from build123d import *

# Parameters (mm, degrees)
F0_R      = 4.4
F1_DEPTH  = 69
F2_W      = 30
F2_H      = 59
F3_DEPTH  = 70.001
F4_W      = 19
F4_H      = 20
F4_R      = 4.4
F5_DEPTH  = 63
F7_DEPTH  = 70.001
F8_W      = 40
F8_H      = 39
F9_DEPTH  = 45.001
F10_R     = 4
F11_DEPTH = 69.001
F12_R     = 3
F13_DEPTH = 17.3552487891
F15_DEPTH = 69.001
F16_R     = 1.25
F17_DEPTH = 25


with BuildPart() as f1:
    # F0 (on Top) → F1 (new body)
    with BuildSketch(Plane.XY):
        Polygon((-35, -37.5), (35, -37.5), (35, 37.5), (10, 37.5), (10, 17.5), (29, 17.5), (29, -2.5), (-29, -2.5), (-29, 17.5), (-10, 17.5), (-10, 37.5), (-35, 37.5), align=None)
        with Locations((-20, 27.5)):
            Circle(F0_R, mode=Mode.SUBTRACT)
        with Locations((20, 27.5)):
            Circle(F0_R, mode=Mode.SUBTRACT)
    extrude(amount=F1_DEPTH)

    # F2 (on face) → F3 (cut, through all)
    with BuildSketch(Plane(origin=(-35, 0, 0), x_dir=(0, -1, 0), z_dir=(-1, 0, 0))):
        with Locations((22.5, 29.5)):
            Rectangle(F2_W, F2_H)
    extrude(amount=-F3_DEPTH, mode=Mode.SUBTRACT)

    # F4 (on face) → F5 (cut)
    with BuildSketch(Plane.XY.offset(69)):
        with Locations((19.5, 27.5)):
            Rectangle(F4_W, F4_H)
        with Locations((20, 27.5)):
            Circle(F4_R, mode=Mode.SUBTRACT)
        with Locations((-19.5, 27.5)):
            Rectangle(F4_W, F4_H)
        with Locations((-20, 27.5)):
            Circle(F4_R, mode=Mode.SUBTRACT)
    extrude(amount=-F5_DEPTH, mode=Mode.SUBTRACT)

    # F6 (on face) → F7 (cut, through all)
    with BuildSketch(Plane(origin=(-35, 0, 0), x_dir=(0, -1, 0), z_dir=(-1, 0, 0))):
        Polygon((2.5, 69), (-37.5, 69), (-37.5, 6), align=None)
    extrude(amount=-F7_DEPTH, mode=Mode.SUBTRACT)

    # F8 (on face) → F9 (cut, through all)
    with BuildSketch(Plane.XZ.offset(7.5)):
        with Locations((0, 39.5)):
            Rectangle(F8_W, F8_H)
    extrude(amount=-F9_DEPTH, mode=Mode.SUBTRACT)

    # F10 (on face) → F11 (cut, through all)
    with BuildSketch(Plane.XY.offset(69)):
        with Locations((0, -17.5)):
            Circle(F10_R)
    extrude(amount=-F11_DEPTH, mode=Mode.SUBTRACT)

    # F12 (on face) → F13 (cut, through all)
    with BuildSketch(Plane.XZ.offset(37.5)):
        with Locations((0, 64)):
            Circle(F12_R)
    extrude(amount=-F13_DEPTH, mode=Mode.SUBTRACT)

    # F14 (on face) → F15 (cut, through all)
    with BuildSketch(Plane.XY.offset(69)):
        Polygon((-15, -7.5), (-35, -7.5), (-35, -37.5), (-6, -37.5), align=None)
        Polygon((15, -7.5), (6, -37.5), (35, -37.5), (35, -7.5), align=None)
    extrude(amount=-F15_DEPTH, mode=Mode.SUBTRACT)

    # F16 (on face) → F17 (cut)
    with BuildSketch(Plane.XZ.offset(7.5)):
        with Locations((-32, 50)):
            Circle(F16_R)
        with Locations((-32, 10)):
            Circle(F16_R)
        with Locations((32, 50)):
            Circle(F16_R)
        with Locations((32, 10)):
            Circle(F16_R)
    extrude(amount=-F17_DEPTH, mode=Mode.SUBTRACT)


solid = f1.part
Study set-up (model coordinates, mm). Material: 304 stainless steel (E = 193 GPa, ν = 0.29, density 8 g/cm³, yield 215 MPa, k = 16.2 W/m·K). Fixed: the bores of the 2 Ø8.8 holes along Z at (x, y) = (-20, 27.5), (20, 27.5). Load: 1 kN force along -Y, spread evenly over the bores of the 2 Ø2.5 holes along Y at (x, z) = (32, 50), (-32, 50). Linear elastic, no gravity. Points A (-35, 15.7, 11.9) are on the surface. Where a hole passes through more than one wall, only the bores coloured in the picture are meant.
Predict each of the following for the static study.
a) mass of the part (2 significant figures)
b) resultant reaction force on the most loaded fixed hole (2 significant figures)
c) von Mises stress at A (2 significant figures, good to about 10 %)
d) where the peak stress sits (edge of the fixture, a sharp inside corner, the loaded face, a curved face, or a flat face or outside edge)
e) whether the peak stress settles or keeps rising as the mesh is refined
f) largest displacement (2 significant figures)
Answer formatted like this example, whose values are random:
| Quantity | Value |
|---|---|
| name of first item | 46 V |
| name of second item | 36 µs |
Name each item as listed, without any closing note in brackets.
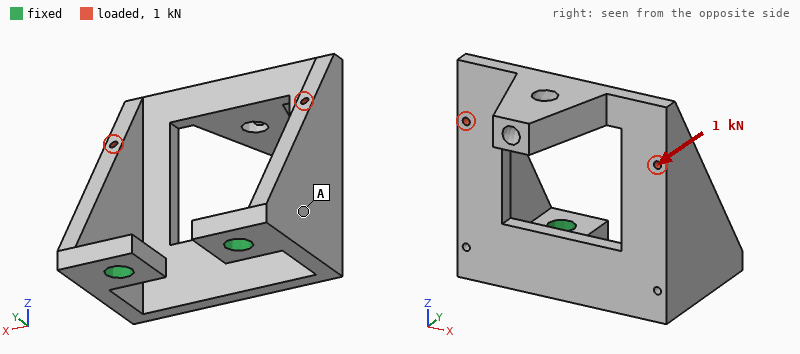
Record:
| Quantity | Value |
|---|---|
| mass of the part | 340 g |
| resultant reaction force on the most loaded fixed hole | 500 N |
| von Mises stress at A | 17 MPa |
| where the peak stress sits | edge of the fixture |
| whether the peak stress settles or keeps rising as the mesh is refined | keeps rising |
| largest displacement | 0.17 mm |
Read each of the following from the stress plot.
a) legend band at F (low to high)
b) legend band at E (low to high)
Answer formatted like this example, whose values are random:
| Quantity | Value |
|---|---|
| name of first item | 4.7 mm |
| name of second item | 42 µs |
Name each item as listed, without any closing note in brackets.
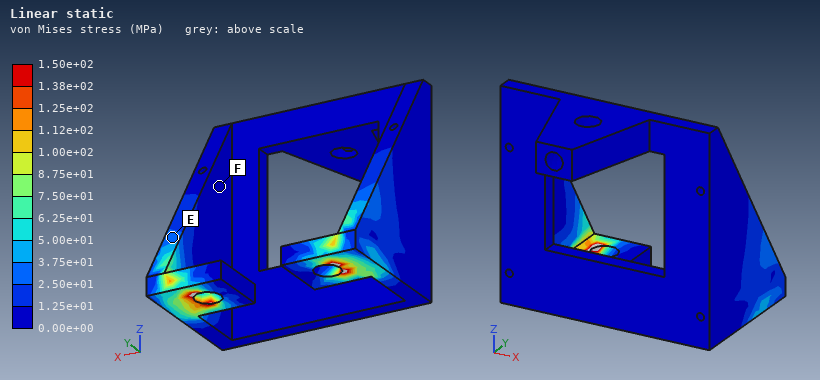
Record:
| Quantity | Value |
|---|---|
| legend band at F | 0.00e+00 to 1.25e+01 MPa |
| legend band at E | 2.50e+01 to 3.75e+01 MPa |
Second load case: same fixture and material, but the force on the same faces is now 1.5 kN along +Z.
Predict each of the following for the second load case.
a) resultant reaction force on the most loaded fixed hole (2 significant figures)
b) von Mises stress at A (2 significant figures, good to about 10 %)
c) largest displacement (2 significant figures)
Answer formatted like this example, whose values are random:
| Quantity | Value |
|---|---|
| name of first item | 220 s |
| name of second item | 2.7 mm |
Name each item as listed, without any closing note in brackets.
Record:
| Quantity | Value |
|---|---|
| resultant reaction force on the most loaded fixed hole | 760 N |
| von Mises stress at A | 16 MPa |
| largest displacement | 0.14 mm |
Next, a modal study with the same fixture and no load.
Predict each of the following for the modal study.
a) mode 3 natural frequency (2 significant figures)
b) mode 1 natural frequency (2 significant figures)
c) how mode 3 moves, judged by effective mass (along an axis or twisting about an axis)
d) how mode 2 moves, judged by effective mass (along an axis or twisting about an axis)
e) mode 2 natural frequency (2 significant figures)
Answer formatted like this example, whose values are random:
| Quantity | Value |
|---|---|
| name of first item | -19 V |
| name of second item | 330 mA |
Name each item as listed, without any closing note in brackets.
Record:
| Quantity | Value |
|---|---|
| mode 3 natural frequency | 2100 Hz |
| mode 1 natural frequency | 930 Hz |
| how mode 3 moves, judged by effective mass | along X |
| how mode 2 moves, judged by effective mass | along X |
| mode 2 natural frequency | 1200 Hz |
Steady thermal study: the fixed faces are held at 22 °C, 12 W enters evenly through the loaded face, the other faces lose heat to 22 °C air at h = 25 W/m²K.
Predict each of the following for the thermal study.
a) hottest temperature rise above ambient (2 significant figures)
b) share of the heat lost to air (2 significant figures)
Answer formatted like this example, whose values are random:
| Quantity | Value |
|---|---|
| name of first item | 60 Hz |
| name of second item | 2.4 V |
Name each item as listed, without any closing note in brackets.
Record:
| Quantity | Value |
|---|---|
| hottest temperature rise above ambient | 56 K |
| share of the heat lost to air | 81 % |
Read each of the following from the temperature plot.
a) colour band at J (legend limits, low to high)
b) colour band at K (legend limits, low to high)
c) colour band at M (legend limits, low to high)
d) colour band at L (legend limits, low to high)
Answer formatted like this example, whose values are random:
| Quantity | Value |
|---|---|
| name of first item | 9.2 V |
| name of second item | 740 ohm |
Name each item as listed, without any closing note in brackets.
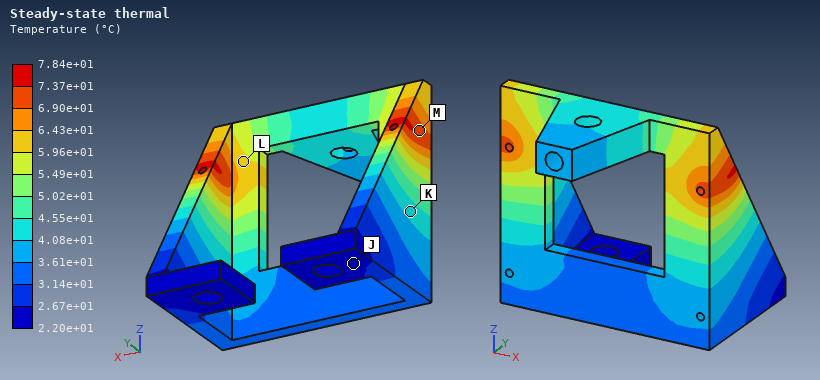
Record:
| Quantity | Value |
|---|---|
| colour band at J | 2.20e+01 to 2.67e+01 °C |
| colour band at K | 4.08e+01 to 4.55e+01 °C |
| colour band at M | 6.90e+01 to 7.37e+01 °C |
| colour band at L | 5.96e+01 to 6.43e+01 °C |
